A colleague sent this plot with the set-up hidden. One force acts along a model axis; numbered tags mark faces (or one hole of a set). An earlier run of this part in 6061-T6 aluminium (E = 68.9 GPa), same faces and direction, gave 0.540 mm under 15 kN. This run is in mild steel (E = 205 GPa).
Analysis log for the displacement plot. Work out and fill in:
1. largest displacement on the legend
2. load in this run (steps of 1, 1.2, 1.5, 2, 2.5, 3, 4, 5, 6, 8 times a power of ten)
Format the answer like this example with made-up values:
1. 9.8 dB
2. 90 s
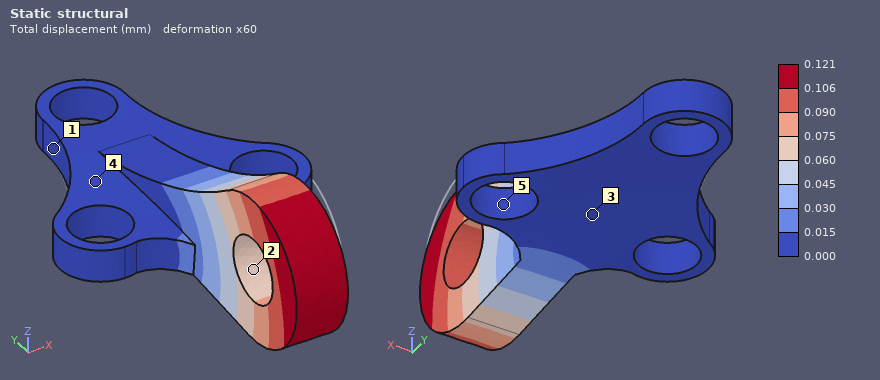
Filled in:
1. 0.121 mm
2. 10 kN
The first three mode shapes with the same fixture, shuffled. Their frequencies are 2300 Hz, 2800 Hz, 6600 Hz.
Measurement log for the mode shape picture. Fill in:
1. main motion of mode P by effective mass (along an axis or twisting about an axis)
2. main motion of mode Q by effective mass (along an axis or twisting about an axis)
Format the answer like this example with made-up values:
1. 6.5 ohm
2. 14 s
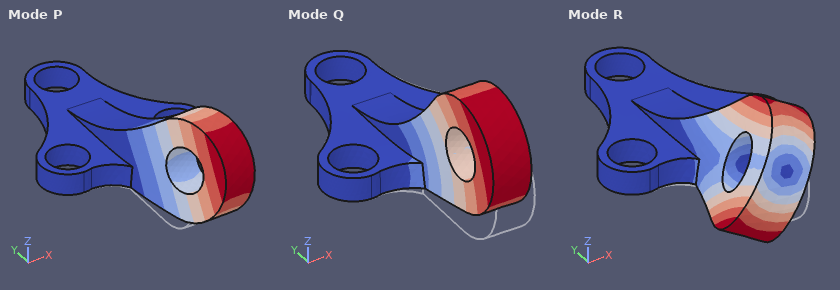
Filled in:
1. along X
2. along Z
